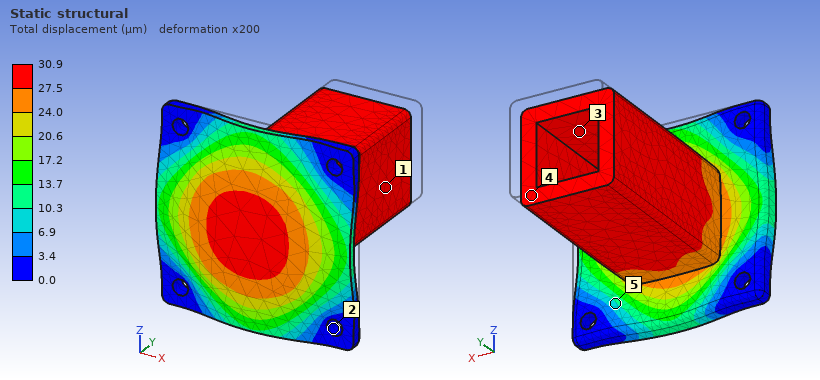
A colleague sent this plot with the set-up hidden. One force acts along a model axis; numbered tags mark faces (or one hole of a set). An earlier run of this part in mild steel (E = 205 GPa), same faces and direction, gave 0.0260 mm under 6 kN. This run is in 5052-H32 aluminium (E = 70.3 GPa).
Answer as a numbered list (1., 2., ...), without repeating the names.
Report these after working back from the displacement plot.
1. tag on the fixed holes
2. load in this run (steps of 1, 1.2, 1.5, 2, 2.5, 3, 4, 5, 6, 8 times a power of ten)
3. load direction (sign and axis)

1. 2
2. 2.5 kN
3. -Y
